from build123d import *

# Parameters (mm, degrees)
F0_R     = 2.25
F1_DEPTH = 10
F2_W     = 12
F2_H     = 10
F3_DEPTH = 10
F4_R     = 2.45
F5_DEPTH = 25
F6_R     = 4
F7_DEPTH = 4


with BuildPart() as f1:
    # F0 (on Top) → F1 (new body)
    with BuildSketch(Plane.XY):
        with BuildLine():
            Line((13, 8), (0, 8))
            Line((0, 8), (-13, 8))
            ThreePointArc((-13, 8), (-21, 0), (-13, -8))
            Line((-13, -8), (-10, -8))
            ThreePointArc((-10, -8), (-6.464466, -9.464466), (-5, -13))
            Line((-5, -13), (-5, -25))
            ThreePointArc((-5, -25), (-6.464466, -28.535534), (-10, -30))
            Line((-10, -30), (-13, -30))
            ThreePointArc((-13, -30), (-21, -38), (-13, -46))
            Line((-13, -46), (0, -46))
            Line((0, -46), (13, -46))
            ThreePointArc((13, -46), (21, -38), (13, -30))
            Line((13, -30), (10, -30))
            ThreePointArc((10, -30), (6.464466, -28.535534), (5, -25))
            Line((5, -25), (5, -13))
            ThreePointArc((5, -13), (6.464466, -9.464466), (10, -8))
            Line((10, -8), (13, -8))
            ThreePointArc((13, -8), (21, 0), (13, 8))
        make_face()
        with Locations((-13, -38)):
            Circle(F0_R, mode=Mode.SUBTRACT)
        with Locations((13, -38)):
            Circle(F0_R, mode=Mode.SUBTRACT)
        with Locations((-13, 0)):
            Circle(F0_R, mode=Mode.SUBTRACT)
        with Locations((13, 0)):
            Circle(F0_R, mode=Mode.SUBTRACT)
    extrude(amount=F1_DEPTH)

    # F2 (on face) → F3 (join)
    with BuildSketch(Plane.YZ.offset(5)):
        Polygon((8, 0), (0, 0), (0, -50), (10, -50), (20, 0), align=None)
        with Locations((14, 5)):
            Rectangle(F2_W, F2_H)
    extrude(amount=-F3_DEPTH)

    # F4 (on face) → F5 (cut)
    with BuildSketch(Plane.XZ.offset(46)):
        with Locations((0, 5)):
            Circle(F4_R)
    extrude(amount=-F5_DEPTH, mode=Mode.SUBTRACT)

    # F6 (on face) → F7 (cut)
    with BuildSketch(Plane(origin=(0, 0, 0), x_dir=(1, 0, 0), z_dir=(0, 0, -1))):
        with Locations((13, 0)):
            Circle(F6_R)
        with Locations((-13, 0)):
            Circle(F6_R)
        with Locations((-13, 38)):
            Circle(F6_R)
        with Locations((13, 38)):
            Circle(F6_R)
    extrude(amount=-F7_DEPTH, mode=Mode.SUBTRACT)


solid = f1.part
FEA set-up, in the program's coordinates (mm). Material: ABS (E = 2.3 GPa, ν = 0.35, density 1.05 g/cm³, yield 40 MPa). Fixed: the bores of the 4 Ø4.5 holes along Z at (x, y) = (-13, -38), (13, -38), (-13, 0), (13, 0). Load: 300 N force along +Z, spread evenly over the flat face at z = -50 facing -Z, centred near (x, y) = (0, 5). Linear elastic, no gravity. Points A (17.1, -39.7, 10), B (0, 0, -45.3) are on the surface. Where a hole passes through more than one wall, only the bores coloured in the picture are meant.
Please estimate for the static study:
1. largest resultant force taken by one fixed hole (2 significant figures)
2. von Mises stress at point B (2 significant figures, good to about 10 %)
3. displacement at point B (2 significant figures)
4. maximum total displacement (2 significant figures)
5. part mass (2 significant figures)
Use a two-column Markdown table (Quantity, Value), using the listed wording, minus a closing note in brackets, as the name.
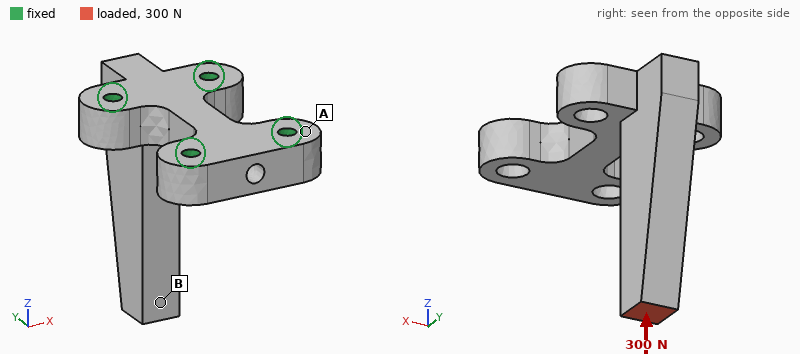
| Quantity | Value |
|---|---|
| largest resultant force taken by one fixed hole | 170 N |
| von Mises stress at point B | 3.3 MPa |
| displacement at point B | 0.13 mm |
| maximum total displacement | 0.13 mm |
| part mass | 23 g |
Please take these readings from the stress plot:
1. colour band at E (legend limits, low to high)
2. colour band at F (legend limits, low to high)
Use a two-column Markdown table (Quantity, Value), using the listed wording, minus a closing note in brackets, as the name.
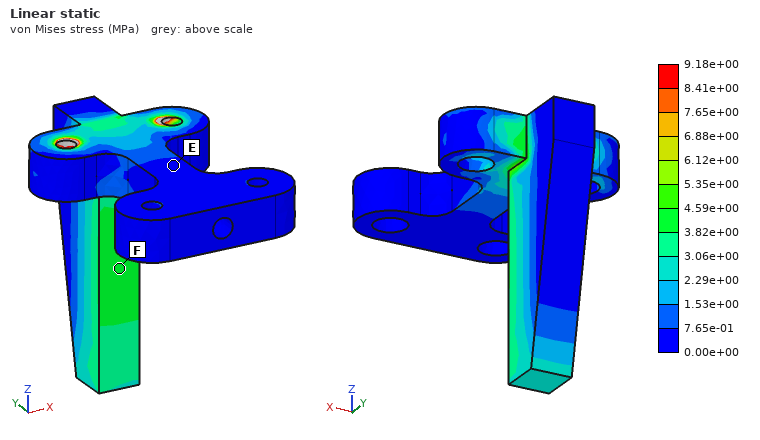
| Quantity | Value |
|---|---|
| colour band at E | 0.00e+00 to 7.65e-01 MPa |
| colour band at F | 3.82e+00 to 4.59e+00 MPa |
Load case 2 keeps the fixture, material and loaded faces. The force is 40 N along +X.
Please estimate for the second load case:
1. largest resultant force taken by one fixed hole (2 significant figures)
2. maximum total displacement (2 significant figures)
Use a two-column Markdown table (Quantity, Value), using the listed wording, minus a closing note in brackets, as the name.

| Quantity | Value |
|---|---|
| largest resultant force taken by one fixed hole | 98 N |
| maximum total displacement | 0.76 mm |
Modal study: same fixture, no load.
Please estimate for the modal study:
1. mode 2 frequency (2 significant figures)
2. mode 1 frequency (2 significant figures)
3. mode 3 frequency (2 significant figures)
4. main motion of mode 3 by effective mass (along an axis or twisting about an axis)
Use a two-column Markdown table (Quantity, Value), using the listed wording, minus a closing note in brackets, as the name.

| Quantity | Value |
|---|---|
| mode 2 frequency | 880 Hz |
| mode 1 frequency | 850 Hz |
| mode 3 frequency | 3700 Hz |
| main motion of mode 3 by effective mass | along Z |
